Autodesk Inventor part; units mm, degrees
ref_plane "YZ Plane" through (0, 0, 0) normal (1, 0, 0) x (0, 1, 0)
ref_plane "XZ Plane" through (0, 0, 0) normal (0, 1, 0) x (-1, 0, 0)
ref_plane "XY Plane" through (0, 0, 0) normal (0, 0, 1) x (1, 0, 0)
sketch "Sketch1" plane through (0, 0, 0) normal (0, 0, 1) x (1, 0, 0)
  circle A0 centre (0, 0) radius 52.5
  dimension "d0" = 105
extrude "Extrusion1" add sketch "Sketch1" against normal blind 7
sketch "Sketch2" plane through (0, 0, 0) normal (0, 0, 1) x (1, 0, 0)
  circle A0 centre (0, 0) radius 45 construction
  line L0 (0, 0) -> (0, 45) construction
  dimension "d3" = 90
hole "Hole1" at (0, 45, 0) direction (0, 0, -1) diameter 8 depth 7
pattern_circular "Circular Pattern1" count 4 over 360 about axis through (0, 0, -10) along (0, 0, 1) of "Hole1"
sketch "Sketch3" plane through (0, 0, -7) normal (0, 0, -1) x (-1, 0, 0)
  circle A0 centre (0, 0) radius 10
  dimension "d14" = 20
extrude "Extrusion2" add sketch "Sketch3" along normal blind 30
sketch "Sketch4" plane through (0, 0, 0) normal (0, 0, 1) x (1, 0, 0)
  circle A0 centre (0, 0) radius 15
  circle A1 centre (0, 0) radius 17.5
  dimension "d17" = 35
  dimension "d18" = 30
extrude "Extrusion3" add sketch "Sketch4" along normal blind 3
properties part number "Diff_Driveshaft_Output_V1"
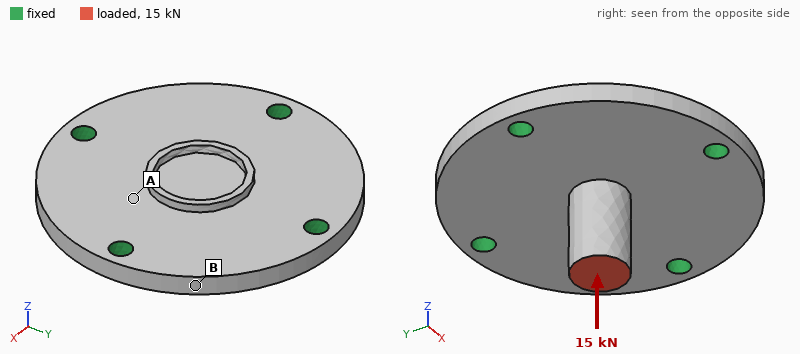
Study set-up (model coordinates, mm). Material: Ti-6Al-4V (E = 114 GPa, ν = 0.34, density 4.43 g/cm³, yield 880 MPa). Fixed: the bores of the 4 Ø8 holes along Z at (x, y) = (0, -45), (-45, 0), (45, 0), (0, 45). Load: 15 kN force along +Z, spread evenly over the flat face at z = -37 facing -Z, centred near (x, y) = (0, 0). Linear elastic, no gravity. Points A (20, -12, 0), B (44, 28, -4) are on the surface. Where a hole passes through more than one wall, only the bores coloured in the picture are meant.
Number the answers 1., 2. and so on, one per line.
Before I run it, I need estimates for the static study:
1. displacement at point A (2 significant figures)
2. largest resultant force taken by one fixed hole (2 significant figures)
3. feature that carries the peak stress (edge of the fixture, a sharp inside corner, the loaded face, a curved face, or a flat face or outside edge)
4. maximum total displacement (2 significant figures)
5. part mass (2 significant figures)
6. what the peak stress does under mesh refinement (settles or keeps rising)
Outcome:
1. 0.084 mm
2. 3.8 kN
3. edge of the fixture
4. 0.15 mm
5. 310 g
6. keeps rising
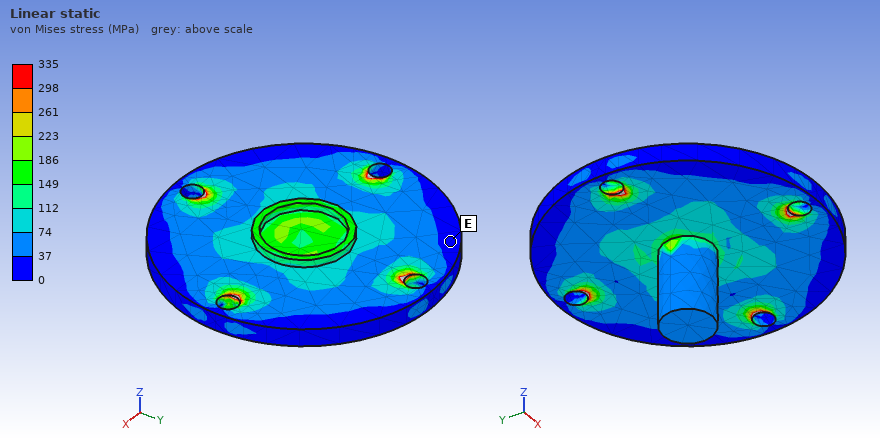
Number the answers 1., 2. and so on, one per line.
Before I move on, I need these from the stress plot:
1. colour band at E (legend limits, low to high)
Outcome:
1. 0 to 37 MPa
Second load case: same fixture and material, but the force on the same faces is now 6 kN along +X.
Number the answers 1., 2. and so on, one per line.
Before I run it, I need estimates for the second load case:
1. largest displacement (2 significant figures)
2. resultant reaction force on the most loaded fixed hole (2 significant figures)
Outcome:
1. 0.25 mm
2. 3.4 kN
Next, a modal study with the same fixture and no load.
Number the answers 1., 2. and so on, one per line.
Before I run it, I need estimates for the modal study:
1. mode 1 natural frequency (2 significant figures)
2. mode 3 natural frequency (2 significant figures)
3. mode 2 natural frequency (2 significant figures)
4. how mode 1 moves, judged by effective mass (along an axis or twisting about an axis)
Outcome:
1. 5300 Hz
2. 6100 Hz
3. 6100 Hz
4. along Z
